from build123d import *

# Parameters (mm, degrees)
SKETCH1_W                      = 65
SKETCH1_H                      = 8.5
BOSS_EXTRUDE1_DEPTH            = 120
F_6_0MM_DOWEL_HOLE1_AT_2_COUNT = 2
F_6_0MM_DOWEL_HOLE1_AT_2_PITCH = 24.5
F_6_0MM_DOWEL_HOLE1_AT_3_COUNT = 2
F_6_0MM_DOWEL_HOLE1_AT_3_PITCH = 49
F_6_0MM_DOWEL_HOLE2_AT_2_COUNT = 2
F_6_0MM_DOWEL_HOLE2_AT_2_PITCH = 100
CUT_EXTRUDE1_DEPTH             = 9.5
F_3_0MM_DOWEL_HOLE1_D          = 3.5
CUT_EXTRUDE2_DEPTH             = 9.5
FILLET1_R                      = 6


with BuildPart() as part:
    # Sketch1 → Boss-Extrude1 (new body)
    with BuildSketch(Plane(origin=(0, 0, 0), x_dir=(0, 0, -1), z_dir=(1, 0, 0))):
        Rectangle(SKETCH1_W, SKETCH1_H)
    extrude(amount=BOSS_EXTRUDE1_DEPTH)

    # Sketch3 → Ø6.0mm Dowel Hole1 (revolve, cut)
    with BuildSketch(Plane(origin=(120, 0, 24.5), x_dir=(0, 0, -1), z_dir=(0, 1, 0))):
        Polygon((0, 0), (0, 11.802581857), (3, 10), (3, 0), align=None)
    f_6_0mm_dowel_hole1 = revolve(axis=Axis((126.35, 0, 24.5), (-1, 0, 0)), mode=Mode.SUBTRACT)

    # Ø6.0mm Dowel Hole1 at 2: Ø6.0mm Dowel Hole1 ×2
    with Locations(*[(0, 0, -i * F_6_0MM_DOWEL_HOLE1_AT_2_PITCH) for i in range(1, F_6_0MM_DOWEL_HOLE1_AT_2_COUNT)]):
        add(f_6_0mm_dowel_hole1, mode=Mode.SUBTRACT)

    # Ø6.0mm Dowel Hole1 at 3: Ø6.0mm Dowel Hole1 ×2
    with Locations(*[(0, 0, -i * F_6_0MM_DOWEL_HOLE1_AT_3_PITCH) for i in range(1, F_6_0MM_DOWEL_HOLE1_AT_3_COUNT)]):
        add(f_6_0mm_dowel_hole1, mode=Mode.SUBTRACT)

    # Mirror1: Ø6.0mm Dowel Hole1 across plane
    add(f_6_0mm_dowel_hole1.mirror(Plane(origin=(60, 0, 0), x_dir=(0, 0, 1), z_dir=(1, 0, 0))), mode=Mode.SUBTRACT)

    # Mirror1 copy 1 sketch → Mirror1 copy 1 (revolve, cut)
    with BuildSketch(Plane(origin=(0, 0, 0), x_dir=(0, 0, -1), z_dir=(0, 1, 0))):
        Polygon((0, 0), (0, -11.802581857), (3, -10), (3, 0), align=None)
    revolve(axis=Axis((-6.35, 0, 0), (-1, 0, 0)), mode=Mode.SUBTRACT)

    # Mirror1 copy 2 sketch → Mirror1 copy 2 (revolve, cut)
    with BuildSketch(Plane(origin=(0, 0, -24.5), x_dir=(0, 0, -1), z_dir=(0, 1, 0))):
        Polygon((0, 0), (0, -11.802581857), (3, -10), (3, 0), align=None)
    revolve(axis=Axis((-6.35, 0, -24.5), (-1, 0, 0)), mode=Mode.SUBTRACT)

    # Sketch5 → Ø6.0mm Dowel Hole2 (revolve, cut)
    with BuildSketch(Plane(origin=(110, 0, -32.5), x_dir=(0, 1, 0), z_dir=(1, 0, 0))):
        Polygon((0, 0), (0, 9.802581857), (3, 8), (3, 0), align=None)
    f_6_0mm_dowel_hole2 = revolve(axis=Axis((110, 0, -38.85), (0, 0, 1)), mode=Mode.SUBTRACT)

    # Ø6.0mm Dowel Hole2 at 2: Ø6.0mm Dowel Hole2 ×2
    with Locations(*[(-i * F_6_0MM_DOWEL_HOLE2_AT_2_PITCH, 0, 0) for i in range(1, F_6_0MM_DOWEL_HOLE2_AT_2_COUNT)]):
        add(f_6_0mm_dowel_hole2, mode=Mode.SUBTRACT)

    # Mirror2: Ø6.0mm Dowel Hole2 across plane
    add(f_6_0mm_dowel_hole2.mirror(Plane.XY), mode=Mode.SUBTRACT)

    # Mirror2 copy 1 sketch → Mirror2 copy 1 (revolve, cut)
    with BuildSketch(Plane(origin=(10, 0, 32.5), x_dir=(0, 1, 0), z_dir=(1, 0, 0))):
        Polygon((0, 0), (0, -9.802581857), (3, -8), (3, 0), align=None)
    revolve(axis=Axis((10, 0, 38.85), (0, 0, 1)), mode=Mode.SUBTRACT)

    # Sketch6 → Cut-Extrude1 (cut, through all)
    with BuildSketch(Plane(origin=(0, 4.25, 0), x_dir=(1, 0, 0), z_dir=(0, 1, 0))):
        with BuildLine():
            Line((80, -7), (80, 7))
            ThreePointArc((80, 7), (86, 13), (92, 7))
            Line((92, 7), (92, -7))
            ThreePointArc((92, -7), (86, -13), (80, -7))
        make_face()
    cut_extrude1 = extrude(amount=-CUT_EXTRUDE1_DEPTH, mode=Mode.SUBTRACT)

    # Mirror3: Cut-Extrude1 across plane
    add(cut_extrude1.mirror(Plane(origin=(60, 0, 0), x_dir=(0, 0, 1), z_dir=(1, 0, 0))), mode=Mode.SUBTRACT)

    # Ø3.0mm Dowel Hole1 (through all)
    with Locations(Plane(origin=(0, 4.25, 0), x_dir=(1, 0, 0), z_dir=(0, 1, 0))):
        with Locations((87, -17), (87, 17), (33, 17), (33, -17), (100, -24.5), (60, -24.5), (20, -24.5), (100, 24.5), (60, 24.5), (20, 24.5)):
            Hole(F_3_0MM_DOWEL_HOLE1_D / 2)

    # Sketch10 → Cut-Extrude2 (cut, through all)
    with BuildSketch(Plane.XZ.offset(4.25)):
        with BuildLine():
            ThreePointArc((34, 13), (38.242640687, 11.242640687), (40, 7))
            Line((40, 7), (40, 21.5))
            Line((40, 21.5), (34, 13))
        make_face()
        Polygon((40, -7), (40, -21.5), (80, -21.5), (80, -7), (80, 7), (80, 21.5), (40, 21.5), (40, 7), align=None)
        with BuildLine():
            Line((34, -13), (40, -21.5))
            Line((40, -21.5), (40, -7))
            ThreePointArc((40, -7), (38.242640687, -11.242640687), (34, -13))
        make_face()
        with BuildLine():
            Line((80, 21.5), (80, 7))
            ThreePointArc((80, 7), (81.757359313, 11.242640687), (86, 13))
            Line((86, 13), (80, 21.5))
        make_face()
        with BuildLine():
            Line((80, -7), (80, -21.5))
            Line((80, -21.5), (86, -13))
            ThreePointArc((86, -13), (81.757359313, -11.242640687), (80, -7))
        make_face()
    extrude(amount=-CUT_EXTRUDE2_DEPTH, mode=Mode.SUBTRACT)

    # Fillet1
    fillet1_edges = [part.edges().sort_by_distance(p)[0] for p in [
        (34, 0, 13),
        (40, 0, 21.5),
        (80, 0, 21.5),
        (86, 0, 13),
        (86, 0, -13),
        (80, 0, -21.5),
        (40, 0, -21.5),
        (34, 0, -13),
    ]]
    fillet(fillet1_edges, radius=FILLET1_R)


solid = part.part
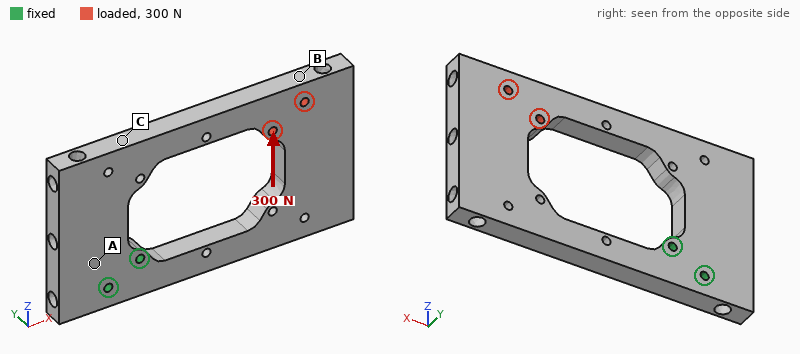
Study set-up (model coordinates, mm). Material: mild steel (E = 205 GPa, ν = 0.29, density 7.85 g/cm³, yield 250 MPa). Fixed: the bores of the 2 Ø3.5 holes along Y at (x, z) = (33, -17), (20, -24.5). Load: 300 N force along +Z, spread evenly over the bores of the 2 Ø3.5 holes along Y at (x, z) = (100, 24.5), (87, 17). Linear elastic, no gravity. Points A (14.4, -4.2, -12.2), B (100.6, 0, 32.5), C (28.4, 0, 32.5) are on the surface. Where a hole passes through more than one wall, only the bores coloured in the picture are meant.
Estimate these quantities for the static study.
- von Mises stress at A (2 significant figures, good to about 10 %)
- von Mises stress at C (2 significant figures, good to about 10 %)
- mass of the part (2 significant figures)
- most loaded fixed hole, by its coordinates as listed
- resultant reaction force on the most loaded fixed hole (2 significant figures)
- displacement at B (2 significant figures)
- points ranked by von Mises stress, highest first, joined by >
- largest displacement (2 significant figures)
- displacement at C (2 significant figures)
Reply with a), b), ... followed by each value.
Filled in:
a) 5.8 MPa
b) 9.0 MPa
c) 330 g
d) (33, -17)
e) 1.4 kN
f) 25 µm
g) C > A > B
h) 28 µm
i) 9.1 µm
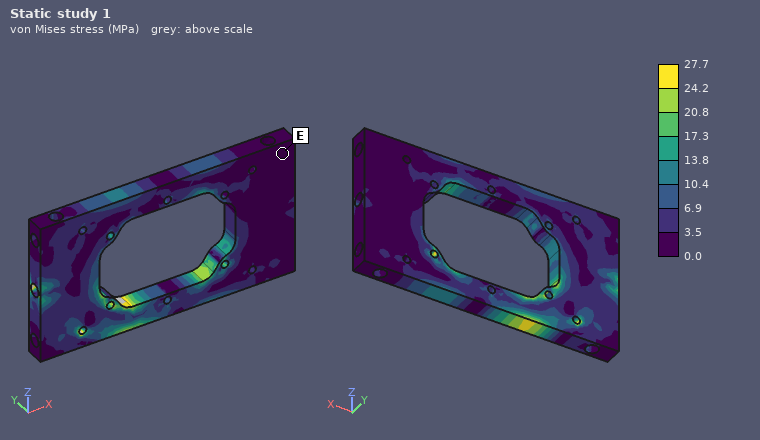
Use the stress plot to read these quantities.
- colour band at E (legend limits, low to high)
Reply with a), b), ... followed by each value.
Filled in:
a) 0.0 to 3.5 MPa
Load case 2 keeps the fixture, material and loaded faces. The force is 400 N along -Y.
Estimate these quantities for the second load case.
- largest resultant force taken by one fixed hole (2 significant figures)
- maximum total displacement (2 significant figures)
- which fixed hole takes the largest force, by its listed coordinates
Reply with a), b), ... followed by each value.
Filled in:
a) 1.7 kN
b) 0.47 mm
c) (33, -17)
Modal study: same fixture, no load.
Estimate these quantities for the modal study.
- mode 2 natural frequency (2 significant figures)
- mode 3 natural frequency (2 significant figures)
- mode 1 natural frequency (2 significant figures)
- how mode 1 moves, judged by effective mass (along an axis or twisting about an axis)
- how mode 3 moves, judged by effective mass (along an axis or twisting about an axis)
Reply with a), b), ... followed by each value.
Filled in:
a) 1300 Hz
b) 1300 Hz
c) 470 Hz
d) along Y
e) along Z
